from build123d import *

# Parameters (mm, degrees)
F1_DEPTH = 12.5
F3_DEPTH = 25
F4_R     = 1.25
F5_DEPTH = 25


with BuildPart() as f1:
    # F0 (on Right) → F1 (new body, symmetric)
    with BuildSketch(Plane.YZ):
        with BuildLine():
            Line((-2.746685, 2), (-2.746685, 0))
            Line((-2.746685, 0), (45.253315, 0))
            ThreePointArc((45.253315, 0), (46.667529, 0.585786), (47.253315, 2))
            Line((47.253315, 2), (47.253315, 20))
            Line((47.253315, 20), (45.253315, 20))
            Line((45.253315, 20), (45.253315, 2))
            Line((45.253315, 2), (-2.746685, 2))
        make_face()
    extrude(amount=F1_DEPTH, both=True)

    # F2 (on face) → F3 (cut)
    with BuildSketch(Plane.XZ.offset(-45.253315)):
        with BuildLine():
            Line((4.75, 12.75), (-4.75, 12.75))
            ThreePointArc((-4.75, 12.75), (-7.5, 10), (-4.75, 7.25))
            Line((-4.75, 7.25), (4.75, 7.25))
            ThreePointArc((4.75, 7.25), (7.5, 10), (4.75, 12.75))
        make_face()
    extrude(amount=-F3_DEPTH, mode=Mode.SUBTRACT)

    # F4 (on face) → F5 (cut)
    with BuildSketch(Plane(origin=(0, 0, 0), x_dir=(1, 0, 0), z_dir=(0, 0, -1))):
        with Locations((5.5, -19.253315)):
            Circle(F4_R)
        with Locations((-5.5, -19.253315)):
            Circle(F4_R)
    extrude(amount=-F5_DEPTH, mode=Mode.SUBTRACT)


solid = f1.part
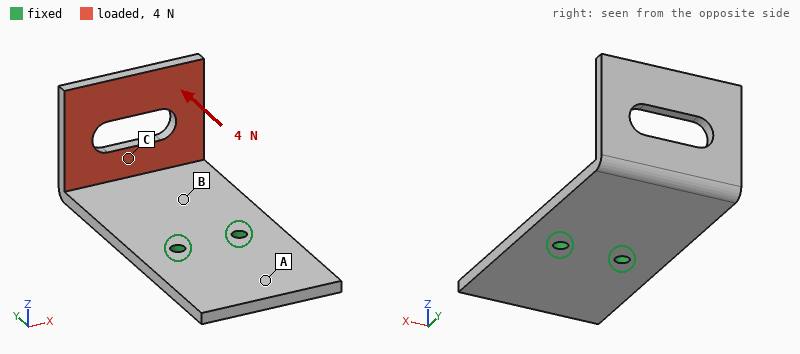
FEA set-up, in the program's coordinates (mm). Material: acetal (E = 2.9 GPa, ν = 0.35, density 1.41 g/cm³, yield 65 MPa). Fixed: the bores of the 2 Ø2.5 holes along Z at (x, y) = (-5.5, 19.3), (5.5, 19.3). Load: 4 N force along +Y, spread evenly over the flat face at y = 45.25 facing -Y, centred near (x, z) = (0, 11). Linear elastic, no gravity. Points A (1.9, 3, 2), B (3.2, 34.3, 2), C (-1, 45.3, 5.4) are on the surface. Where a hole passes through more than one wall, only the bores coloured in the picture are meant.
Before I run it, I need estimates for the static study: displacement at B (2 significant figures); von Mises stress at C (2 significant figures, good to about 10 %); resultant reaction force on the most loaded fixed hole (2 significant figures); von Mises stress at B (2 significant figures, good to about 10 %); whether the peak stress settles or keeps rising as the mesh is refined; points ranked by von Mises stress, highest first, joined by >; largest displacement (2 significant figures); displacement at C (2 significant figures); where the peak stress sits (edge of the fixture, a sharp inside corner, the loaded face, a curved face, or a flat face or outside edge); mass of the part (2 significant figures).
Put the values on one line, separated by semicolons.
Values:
0.093 mm; 0.83 MPa; 2.0 N; 2.3 MPa; keeps rising; B > C > A; 0.62 mm; 0.28 mm; edge of the fixture; 4.5 g
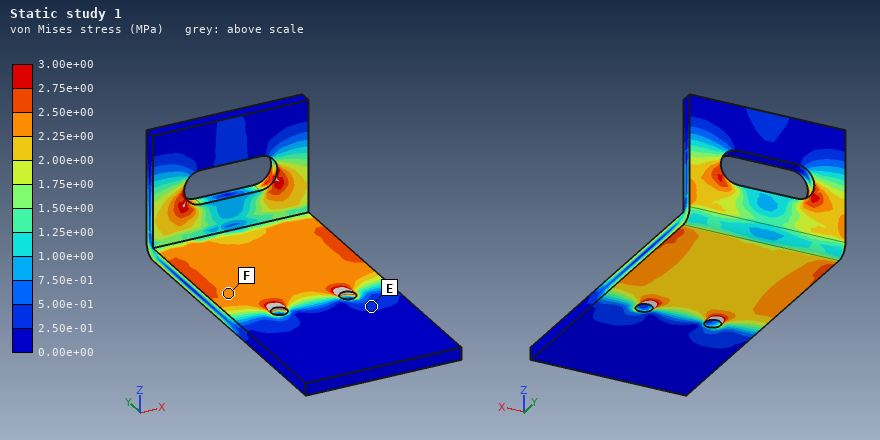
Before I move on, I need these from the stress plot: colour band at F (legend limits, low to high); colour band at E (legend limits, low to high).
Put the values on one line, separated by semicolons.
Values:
2.25e+00 to 2.50e+00 MPa; 2.50e-01 to 5.00e-01 MPa
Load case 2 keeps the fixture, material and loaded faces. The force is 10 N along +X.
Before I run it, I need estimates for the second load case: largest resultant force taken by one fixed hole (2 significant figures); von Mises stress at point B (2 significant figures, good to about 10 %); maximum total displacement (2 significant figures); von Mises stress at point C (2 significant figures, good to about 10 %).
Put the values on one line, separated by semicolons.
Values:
22 N; 5.3 MPa; 0.68 mm; 2.7 MPa
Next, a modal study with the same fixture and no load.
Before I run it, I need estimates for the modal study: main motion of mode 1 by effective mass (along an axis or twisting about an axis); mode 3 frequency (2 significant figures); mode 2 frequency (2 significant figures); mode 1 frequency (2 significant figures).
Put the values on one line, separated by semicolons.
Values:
along Z; 870 Hz; 610 Hz; 310 Hz
